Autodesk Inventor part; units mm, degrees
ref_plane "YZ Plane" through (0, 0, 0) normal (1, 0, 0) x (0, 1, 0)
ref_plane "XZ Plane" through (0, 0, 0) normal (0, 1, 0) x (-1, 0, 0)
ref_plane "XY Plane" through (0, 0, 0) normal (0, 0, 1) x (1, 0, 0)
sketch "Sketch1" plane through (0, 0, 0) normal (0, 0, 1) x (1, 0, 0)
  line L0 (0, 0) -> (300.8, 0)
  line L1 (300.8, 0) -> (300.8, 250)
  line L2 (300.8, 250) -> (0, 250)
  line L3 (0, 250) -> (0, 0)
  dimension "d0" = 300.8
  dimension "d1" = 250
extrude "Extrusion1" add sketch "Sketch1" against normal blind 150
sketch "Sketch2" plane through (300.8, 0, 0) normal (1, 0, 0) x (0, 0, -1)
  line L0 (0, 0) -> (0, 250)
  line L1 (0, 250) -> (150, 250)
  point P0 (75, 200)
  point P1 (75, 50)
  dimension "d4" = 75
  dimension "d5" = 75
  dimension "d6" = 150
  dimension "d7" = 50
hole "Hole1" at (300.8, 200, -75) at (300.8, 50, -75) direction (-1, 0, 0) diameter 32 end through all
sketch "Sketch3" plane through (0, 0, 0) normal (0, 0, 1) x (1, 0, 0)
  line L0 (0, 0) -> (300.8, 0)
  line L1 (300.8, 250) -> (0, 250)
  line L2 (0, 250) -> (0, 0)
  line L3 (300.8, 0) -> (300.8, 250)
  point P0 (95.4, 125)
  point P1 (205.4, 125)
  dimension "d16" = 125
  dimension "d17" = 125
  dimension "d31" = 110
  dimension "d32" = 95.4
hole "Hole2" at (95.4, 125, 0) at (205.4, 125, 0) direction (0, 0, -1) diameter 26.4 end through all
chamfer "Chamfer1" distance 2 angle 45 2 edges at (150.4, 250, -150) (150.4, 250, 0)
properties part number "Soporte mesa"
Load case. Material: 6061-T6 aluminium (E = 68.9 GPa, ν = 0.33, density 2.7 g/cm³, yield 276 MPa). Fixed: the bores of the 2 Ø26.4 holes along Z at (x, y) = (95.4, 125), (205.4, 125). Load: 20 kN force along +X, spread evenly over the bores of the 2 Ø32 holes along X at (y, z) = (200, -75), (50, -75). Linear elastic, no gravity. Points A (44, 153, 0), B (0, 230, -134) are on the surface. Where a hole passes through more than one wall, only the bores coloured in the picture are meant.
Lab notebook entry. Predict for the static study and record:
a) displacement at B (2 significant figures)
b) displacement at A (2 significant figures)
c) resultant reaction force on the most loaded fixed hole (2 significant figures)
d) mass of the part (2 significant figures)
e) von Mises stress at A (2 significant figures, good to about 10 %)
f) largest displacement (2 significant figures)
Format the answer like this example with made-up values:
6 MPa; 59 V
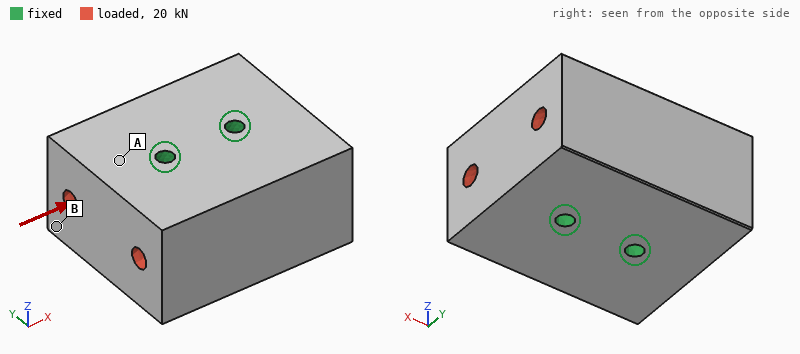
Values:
0.94 µm; 0.34 µm; 10 kN; 29 kg; 0.34 MPa; 1.3 µm
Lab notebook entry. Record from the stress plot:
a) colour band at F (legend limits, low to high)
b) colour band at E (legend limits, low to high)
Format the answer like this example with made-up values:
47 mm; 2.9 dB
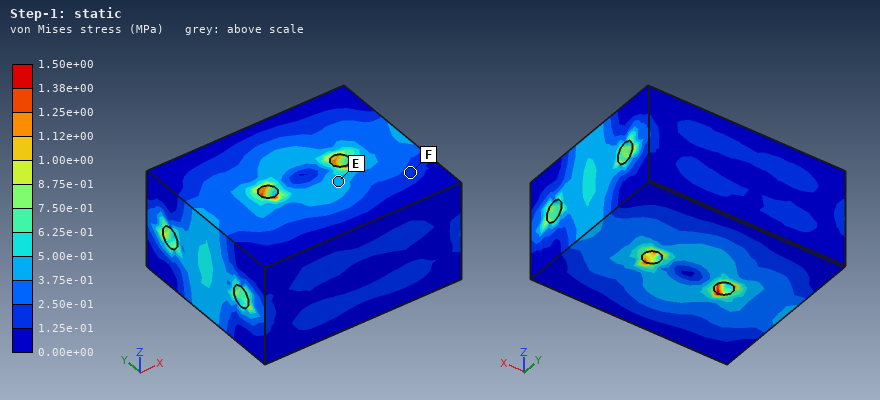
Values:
1.25e-01 to 2.50e-01 MPa; 3.75e-01 to 5.00e-01 MPa
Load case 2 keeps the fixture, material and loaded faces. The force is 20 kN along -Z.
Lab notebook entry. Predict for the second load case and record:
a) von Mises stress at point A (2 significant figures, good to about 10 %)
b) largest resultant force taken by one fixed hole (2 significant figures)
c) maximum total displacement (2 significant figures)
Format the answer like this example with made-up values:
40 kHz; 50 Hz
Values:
0.41 MPa; 10 kN; 1.8 µm
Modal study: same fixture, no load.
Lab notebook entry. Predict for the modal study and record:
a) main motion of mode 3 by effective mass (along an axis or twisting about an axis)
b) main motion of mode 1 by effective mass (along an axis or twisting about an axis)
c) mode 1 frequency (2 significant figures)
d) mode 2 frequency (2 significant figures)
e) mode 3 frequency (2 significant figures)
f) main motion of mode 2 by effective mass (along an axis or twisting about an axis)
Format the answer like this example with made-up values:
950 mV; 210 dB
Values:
twisting about Y; twisting about Z; 2800 Hz; 3300 Hz; 3800 Hz; twisting about X
